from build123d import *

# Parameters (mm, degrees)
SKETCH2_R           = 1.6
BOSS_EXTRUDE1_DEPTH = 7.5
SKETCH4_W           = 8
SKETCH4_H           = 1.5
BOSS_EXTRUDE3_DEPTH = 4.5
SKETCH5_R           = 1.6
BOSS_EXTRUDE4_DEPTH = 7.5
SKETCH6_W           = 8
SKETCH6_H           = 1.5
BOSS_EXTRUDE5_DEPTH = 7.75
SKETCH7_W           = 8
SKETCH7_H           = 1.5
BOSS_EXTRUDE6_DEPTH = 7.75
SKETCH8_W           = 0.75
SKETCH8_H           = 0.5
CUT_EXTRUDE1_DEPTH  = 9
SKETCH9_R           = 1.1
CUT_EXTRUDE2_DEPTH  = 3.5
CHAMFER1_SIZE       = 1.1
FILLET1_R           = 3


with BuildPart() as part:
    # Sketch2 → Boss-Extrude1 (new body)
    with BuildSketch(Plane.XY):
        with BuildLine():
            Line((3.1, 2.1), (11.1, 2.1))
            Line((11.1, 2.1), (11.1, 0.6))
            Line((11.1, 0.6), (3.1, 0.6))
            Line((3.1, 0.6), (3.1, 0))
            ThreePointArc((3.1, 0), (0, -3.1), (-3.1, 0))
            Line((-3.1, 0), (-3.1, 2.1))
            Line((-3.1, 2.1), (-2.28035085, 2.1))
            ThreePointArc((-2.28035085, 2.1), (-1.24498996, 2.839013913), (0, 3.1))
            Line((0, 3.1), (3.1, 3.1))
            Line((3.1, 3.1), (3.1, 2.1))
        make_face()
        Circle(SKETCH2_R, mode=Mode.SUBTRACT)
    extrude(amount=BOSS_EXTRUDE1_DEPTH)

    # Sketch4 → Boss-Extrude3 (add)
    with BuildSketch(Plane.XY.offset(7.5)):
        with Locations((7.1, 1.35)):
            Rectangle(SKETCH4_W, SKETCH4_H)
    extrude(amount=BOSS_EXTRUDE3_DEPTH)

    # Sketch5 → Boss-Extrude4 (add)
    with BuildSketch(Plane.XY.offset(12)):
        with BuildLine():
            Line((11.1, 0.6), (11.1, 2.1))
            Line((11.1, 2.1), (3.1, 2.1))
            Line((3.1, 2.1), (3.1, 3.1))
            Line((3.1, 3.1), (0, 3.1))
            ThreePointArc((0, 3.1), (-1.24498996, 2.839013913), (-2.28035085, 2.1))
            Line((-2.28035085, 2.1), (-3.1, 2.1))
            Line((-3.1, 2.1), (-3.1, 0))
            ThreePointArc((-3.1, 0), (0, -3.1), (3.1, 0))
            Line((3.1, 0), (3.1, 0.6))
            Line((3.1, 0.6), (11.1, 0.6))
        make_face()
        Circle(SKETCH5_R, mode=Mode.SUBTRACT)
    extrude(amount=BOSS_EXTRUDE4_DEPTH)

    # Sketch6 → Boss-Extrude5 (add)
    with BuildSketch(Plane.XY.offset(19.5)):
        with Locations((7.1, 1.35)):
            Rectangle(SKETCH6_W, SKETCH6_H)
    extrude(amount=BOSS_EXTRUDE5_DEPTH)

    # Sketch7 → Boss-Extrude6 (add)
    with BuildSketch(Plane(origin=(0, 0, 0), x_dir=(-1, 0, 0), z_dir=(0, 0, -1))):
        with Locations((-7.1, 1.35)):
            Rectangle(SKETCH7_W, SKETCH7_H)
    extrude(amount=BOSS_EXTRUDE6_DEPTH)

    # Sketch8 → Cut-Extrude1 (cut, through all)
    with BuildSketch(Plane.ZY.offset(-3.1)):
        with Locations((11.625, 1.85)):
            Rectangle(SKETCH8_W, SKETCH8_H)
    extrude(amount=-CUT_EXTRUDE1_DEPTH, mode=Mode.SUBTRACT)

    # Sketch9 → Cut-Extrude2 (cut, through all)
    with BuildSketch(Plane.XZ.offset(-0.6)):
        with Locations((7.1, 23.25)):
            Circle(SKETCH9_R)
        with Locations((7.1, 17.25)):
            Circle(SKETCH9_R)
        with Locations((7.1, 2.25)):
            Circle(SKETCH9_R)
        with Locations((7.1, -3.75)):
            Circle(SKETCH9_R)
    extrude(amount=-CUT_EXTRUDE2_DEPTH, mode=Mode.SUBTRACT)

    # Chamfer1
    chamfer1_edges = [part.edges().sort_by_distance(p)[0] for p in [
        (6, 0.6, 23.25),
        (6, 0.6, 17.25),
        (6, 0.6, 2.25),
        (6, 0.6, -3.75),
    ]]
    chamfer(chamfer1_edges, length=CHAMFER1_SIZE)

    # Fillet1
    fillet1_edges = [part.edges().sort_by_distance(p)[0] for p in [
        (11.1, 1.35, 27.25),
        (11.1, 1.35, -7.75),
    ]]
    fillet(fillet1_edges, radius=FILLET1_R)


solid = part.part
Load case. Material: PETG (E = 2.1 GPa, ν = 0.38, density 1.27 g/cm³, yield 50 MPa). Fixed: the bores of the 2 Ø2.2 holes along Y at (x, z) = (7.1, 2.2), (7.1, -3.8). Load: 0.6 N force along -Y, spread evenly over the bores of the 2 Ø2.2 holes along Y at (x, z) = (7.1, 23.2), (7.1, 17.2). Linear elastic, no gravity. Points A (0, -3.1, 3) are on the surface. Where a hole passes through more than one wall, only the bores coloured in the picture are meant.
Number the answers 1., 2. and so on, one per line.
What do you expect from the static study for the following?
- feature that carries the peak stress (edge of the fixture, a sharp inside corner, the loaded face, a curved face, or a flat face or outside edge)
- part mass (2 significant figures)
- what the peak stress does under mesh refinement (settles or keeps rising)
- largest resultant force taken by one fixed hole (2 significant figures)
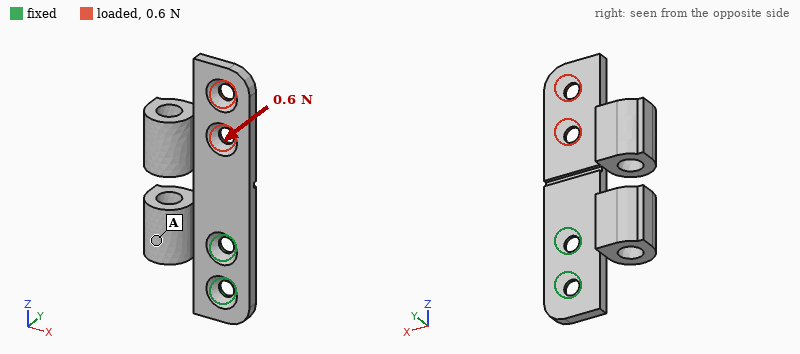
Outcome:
1. edge of the fixture
2. 0.94 g
3. keeps rising
4. 3.1 N
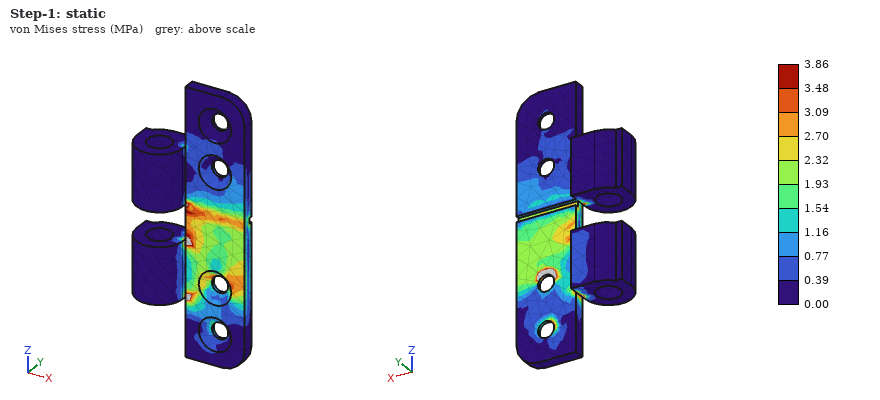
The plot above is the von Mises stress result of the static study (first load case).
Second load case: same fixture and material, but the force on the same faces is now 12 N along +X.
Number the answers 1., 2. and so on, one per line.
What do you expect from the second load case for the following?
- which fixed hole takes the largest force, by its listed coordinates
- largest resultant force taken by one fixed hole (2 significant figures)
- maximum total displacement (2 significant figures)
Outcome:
1. (7.1, 2.2)
2. 37 N
3. 0.44 mm
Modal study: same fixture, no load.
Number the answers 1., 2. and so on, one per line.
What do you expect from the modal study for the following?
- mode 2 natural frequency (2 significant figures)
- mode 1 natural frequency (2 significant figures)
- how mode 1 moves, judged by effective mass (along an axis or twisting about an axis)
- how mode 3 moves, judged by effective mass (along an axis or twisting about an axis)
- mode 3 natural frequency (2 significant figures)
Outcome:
1. 910 Hz
2. 430 Hz
3. along Y
4. along X
5. 1700 Hz
